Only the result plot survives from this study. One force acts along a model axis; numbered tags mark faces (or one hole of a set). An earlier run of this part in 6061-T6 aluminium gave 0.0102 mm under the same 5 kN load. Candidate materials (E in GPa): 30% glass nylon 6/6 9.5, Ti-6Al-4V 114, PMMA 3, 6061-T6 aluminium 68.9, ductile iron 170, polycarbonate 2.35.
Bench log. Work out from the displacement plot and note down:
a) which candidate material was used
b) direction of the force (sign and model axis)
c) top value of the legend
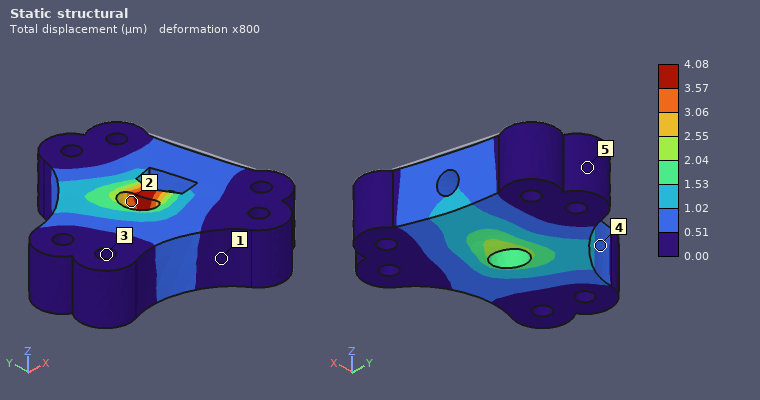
ductile iron
-X
4.08 µm
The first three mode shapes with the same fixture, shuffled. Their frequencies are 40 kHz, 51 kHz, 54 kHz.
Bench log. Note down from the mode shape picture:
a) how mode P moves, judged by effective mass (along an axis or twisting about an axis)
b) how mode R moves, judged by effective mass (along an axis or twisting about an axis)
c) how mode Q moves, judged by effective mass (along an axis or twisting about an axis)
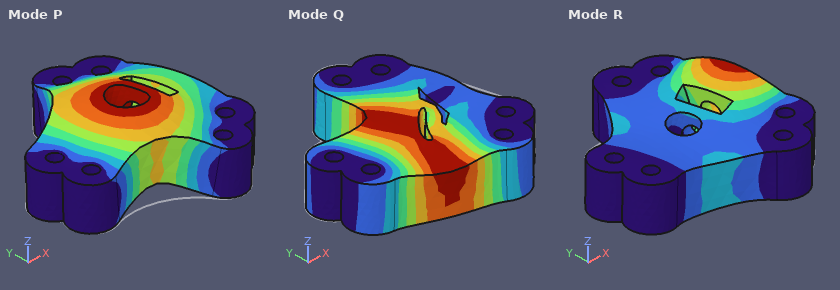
along Z
twisting about Y
along Y
